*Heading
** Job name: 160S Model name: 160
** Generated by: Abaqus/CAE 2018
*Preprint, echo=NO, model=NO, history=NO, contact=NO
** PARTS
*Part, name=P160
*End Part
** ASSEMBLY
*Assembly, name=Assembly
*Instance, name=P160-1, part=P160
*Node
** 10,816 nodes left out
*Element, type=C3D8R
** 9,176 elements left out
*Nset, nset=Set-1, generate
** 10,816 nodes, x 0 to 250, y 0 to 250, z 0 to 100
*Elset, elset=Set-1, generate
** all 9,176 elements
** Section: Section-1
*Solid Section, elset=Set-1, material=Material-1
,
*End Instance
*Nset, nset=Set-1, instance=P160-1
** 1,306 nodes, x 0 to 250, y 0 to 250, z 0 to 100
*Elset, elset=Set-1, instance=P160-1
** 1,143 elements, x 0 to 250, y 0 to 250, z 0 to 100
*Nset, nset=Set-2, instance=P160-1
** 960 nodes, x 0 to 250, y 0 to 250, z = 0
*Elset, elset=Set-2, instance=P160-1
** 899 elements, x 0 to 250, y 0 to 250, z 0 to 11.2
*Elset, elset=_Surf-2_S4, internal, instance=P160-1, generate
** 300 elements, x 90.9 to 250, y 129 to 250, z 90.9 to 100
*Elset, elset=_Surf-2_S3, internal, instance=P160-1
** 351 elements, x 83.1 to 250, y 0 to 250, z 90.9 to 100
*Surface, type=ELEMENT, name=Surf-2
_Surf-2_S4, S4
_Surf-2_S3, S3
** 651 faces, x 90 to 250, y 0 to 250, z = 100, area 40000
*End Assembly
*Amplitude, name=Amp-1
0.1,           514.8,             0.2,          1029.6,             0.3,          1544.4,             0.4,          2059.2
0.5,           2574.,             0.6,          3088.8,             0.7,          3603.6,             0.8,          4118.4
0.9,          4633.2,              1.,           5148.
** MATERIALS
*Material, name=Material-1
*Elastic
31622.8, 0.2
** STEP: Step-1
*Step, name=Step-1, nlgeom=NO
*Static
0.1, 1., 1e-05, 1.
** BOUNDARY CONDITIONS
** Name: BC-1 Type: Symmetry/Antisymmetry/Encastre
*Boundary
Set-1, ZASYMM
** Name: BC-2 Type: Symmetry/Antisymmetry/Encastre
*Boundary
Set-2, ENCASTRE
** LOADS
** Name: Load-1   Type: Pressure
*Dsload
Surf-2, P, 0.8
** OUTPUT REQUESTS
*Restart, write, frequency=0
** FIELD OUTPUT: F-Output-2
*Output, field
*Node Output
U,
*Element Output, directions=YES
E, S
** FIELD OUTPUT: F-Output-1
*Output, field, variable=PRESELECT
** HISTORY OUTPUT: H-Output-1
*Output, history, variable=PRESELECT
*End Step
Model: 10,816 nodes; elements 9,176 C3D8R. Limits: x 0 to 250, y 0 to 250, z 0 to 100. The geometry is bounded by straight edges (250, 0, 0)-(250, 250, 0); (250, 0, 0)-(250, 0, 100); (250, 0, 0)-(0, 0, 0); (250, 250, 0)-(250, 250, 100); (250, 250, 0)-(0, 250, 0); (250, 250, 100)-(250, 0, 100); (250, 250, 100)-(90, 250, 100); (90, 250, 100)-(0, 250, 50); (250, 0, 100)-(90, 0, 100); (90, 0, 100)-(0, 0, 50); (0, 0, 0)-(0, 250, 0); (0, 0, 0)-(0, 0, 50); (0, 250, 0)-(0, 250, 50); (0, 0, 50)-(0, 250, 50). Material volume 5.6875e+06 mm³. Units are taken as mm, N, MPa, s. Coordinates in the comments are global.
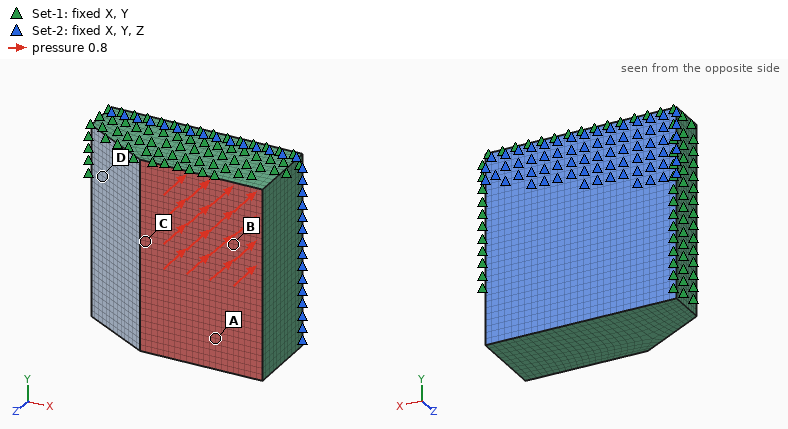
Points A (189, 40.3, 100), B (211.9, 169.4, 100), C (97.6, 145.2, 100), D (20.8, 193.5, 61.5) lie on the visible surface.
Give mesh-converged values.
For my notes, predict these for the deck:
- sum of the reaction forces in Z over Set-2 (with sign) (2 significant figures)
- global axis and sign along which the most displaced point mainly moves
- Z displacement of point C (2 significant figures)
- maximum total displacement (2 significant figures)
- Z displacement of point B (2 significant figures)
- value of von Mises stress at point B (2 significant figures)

32000 N
-Z
-0.0015 mm
0.0023 mm
-0.0023 mm
0.58 MPa
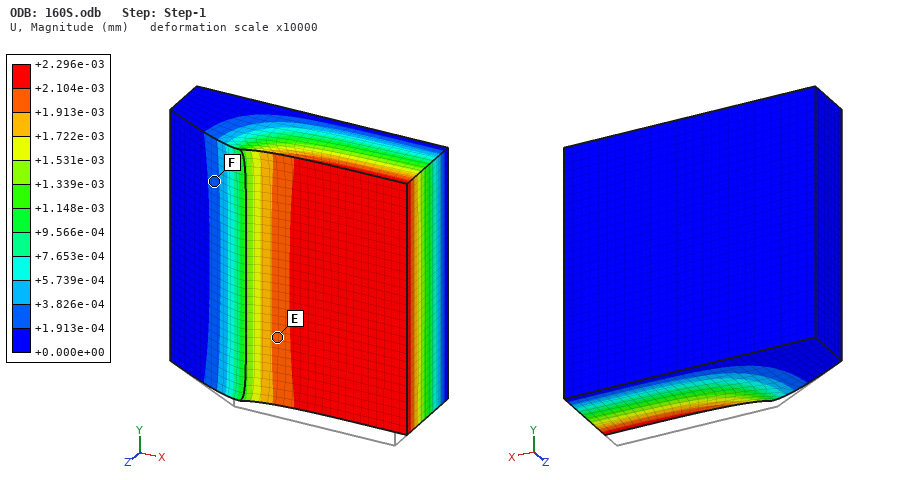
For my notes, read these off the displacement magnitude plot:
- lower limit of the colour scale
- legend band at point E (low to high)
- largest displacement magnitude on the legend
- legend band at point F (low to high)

+0.000e+00 mm
+1.913e-03 to +2.104e-03 mm
+2.296e-03 mm
+1.913e-04 to +3.826e-04 mm
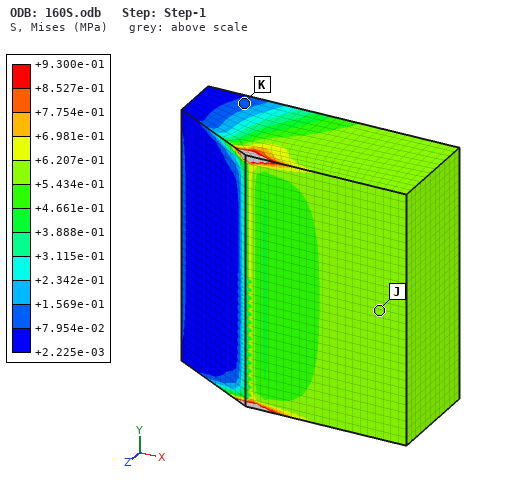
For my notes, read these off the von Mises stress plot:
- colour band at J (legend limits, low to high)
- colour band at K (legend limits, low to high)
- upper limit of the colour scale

+5.434e-01 to +6.207e-01 MPa
+7.954e-02 to +1.569e-01 MPa
+9.300e-01 MPa
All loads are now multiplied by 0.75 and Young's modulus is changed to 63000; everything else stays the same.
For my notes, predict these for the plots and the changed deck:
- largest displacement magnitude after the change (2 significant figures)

8.6e-04 mm
